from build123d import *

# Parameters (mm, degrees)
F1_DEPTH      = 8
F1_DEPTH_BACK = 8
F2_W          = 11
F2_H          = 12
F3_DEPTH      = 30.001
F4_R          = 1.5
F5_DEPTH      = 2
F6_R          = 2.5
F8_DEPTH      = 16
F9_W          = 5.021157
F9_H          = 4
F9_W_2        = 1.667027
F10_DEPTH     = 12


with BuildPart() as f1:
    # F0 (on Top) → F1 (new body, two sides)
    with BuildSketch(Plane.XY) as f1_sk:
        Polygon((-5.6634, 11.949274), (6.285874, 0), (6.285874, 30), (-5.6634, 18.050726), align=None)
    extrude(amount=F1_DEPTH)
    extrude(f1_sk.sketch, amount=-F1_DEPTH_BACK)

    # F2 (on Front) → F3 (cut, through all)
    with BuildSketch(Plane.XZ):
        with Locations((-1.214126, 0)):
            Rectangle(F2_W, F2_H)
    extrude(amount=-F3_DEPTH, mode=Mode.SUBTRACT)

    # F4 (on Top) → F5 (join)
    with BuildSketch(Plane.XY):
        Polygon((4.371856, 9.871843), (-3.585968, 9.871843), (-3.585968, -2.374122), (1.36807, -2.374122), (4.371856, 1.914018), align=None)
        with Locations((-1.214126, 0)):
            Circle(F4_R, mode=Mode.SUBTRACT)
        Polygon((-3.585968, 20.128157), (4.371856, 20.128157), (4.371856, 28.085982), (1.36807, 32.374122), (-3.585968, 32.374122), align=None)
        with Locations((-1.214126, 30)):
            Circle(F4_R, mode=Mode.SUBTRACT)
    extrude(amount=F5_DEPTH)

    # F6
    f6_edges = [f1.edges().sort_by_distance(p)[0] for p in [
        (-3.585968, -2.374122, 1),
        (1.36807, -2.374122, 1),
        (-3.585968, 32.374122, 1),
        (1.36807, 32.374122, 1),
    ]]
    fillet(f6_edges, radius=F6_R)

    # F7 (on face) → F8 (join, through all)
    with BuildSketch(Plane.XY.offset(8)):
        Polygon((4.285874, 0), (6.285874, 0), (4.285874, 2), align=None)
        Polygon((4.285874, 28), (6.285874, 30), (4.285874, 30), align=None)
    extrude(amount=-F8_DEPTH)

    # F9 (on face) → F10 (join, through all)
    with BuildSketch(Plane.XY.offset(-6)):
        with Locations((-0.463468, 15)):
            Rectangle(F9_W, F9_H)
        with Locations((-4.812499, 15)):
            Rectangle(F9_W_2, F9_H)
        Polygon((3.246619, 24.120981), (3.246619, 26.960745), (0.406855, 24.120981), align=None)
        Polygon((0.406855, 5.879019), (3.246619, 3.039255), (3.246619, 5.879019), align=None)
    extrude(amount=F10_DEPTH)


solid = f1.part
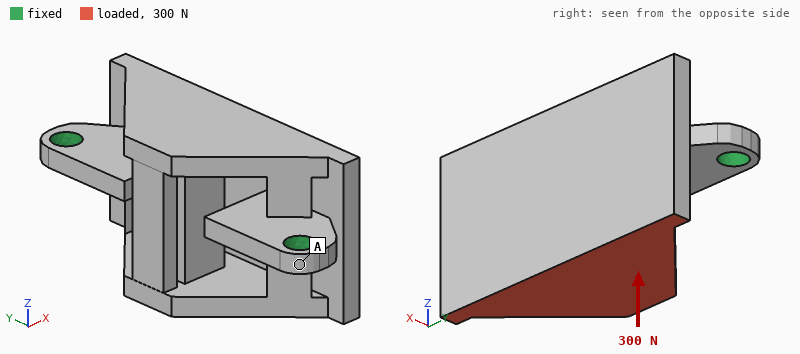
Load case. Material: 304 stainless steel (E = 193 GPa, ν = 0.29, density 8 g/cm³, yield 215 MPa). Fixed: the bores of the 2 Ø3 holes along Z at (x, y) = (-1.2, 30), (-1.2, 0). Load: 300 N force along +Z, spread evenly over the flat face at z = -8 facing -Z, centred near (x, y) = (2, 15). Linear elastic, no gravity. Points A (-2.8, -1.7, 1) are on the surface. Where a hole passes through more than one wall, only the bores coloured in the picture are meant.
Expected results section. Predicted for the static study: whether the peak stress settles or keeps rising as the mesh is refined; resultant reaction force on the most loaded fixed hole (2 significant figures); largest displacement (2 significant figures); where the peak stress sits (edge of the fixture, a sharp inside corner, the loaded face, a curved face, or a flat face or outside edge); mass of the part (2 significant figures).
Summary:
keeps rising
150 N
5.2 µm
edge of the fixture
19 g
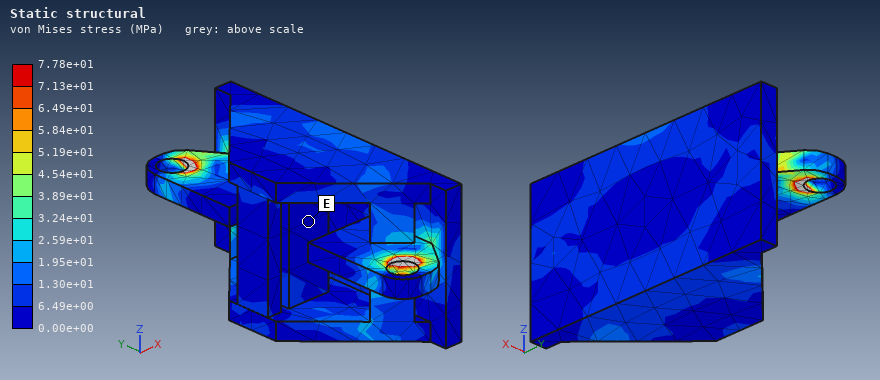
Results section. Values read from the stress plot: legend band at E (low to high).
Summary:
0.00e+00 to 6.49e+00 MPa
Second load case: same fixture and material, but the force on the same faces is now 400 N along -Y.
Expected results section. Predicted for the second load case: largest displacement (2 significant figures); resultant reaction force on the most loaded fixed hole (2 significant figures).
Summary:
11 µm
240 N
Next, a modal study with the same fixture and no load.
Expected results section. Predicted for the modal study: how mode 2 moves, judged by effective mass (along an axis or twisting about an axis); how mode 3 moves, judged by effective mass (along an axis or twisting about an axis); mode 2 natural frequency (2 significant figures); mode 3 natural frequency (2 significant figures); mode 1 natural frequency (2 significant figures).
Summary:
along Z
along Y
10 kHz
13 kHz
4300 Hz
